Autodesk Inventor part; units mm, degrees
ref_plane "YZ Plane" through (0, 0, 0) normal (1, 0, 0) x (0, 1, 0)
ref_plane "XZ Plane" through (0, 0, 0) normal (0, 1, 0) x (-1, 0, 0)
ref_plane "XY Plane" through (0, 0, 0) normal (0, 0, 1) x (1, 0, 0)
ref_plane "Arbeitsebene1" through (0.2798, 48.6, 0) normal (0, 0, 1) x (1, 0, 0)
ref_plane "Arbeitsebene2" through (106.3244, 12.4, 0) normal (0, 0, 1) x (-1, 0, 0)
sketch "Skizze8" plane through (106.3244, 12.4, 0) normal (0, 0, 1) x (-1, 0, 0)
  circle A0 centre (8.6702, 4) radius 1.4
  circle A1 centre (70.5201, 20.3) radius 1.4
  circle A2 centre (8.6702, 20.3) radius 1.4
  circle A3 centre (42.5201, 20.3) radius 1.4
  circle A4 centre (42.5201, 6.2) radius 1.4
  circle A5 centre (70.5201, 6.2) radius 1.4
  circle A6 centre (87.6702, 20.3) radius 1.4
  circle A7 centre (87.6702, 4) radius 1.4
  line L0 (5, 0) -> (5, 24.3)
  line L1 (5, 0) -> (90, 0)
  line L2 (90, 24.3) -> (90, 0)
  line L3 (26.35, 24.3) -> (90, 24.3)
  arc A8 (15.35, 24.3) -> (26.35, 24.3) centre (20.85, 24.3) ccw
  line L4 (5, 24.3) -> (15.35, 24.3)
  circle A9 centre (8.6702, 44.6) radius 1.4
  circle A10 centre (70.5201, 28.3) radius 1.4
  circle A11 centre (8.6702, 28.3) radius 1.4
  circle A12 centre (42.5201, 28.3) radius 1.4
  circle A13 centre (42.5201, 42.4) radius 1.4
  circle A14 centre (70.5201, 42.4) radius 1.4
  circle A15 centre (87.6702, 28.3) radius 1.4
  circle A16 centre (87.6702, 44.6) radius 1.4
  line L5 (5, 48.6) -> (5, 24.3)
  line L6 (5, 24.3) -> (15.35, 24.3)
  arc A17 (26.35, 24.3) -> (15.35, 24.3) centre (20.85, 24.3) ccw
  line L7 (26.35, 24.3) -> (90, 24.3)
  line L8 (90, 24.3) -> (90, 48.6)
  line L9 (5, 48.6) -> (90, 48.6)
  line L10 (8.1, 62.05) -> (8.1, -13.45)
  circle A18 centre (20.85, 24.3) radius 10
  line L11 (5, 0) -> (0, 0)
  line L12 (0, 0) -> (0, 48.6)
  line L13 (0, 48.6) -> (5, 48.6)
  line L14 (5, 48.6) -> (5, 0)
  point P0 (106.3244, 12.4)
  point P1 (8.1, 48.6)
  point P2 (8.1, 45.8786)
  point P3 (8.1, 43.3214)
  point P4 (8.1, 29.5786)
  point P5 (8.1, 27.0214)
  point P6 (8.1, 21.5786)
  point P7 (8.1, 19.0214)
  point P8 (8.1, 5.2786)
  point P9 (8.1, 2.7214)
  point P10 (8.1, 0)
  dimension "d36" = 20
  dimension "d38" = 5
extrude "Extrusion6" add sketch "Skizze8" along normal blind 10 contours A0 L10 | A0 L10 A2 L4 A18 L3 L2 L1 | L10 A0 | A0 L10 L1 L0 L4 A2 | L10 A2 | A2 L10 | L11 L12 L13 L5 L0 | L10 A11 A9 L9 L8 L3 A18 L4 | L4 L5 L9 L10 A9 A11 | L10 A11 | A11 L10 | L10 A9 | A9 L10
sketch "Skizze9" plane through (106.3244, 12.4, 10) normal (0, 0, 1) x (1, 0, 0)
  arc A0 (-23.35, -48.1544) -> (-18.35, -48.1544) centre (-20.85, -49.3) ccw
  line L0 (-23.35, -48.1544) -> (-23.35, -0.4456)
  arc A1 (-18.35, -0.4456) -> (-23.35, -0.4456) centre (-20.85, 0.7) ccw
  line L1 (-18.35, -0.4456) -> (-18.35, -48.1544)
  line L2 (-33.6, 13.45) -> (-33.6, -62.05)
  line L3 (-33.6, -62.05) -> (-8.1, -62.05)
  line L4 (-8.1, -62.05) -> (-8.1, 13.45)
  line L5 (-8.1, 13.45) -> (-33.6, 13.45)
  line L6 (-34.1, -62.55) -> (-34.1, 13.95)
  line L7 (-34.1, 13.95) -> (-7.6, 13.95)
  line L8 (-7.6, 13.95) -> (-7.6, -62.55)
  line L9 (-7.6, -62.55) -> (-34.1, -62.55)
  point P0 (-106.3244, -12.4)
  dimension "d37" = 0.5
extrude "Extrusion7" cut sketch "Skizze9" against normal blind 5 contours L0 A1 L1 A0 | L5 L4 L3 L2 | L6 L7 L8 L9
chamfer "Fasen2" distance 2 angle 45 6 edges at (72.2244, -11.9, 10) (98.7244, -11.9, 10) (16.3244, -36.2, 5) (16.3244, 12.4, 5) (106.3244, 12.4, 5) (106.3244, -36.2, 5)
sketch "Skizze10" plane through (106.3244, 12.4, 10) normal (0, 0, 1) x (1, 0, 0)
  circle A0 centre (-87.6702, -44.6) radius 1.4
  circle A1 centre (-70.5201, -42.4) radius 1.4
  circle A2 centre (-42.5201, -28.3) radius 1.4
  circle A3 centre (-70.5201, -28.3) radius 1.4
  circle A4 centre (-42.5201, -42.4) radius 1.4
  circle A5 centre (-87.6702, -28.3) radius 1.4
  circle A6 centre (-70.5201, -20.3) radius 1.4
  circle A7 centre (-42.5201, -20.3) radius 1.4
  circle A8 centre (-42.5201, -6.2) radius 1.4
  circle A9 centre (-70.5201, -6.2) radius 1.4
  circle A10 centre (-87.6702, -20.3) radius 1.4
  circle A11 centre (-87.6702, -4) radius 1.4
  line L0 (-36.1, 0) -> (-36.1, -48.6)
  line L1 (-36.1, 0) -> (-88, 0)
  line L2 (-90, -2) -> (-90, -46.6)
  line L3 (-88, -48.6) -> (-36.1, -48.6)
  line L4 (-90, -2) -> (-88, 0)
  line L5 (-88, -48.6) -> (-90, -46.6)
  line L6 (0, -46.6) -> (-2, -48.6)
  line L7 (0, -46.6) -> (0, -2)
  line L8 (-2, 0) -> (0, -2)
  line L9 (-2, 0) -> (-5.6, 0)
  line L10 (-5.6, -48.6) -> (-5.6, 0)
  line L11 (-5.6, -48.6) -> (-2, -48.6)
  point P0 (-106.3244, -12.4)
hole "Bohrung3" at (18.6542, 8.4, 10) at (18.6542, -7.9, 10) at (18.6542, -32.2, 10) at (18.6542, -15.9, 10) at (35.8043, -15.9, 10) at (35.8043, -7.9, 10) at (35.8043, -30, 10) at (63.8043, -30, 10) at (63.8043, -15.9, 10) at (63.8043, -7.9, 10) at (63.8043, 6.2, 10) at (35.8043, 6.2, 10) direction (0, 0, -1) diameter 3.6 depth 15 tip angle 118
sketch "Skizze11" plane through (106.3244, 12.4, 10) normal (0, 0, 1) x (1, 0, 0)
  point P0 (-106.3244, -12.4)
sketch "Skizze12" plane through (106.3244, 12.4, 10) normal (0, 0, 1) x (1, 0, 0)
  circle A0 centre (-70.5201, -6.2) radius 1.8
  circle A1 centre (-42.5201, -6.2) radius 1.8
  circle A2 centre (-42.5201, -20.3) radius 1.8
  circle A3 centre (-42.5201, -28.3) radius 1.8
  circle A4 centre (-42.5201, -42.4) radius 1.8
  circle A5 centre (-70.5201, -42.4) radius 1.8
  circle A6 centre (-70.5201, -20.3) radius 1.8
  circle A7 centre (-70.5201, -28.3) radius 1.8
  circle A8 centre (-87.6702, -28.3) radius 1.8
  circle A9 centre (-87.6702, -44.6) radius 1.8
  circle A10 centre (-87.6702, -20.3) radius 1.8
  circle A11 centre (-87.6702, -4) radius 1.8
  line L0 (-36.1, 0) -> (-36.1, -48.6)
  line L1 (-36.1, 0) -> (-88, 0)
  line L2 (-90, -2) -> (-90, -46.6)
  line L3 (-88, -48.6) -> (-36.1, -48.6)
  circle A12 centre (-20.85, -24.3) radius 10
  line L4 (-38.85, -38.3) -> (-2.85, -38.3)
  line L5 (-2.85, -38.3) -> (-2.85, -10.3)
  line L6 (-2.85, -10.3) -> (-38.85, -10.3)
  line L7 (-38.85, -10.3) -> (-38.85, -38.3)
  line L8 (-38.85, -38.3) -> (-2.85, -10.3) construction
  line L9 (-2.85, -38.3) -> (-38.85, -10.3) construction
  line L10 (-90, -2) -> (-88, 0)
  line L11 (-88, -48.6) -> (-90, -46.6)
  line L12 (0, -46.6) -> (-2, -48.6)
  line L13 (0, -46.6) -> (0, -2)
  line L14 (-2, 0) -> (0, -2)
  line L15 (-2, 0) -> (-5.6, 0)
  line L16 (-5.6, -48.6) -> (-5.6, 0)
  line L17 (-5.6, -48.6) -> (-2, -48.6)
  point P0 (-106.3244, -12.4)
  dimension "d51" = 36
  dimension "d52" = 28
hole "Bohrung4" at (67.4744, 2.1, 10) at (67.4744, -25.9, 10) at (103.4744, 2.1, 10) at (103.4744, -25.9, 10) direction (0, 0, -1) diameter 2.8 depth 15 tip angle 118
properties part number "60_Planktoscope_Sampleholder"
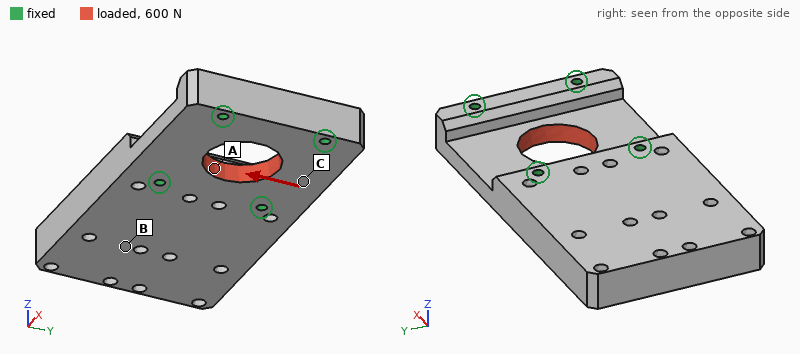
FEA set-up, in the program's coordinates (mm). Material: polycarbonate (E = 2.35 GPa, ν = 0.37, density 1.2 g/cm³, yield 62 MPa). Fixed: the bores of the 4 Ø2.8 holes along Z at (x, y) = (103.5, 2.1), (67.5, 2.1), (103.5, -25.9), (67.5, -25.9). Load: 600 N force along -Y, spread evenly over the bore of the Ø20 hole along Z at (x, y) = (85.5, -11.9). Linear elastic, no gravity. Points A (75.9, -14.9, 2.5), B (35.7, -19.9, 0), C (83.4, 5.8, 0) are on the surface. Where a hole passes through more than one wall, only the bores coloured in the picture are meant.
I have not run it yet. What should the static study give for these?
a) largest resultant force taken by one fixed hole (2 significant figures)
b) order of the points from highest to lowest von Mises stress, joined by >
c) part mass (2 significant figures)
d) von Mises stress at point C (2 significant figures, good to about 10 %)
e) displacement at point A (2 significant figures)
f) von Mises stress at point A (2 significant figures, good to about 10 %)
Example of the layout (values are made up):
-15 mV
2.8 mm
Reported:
160 N
A > C > B
41 g
1.4 MPa
17 µm
3.7 MPa
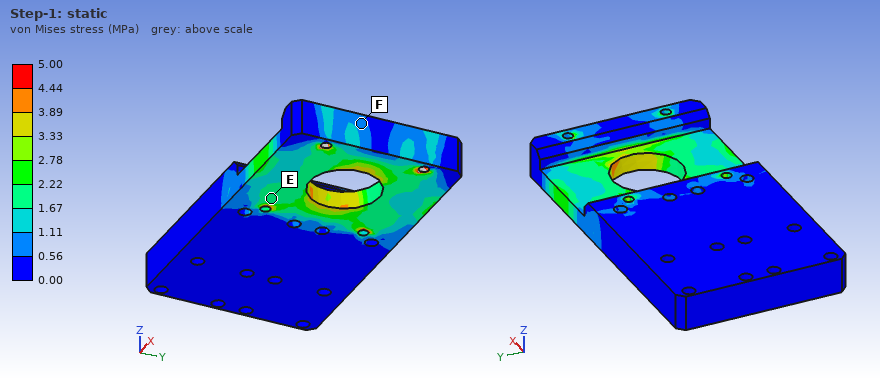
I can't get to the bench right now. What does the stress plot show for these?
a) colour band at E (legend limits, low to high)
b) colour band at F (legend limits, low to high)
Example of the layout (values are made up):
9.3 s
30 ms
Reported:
1.67 to 2.22 MPa
0.56 to 1.11 MPa
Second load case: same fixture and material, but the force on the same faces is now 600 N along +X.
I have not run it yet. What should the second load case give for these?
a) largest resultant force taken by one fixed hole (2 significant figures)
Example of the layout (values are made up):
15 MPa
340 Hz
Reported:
160 N
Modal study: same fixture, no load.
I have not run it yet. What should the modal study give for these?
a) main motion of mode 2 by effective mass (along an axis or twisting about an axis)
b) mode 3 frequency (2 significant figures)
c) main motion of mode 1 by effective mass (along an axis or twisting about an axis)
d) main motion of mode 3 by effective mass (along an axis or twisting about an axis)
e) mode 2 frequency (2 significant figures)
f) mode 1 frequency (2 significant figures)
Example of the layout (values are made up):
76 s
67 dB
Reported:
twisting about X
2300 Hz
along Z
along Y
1800 Hz
720 Hz
